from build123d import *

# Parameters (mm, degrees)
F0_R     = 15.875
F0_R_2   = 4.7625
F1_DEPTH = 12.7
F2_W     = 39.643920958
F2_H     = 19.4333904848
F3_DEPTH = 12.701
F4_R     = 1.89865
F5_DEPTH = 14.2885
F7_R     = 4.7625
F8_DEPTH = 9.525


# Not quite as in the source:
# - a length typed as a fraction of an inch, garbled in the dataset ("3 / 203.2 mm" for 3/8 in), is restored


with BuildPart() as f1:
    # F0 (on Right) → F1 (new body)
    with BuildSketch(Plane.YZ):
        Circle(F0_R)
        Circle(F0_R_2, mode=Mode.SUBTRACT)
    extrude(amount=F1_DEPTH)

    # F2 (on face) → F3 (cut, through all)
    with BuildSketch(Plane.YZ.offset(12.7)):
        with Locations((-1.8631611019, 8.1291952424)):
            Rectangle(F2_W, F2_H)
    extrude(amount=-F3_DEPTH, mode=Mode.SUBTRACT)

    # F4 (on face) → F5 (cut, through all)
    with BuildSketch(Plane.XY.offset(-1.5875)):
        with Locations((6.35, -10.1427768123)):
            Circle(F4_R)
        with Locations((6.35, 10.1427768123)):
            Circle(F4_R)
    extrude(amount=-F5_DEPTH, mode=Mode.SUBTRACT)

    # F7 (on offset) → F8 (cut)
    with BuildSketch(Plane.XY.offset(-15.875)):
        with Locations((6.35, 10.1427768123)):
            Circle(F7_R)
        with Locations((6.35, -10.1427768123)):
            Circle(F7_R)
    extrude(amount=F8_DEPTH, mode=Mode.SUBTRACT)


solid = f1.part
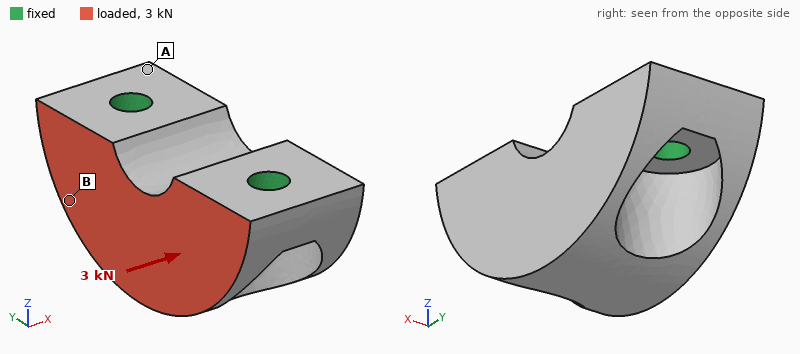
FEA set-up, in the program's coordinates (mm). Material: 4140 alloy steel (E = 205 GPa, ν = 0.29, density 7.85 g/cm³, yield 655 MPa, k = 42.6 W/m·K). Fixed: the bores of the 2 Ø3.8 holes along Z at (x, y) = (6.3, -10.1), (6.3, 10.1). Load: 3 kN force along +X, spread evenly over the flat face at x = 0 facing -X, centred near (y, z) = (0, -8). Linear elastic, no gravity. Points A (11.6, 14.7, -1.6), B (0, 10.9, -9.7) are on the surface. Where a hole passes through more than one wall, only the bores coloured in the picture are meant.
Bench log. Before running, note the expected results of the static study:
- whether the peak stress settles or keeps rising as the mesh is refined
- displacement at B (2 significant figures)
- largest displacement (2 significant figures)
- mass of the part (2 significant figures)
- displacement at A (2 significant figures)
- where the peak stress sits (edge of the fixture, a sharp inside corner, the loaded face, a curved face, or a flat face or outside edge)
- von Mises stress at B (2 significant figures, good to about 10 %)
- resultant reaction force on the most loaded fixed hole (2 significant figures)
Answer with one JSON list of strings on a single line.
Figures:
["keeps rising", "6.9 µm", "11 µm", "25 g", "1.7 µm", "edge of the fixture", "31 MPa", "1.5 kN"]
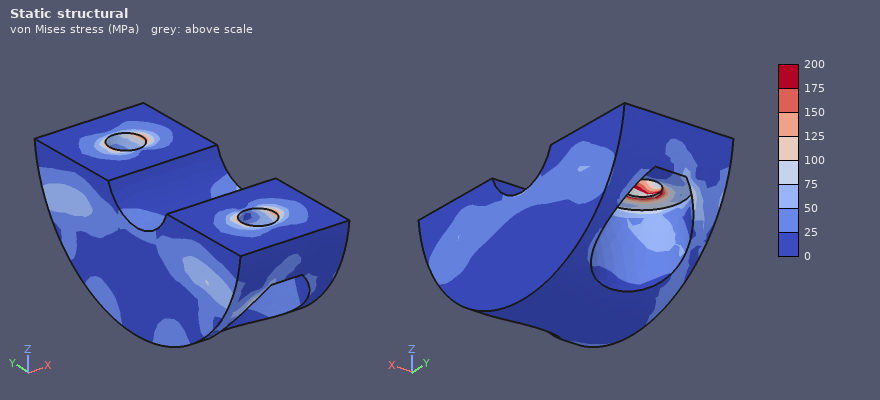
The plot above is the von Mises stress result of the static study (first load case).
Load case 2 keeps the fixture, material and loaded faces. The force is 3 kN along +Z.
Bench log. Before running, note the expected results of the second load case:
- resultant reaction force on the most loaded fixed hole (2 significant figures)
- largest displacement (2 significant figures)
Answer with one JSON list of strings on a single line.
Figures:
["1.6 kN", "13 µm"]
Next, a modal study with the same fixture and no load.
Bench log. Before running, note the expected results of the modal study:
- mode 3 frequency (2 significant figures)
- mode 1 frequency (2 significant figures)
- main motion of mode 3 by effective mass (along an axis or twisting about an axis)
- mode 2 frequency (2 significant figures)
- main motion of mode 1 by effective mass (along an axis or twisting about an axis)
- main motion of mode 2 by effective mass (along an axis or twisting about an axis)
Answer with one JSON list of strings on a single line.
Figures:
["44 kHz", "20 kHz", "along Y", "41 kHz", "along X", "along Z"]
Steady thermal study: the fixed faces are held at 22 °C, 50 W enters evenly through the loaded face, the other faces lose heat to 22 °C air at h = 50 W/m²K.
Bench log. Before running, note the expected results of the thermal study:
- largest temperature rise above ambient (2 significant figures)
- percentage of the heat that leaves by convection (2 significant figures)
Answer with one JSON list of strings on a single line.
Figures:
["68 K", "4.3 %"]
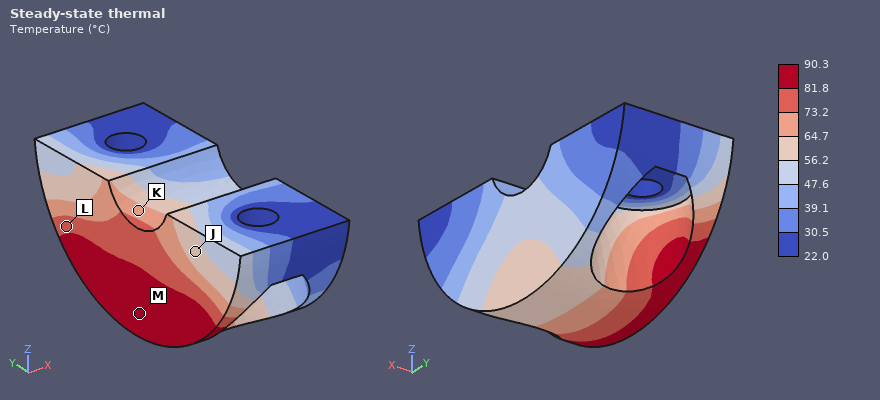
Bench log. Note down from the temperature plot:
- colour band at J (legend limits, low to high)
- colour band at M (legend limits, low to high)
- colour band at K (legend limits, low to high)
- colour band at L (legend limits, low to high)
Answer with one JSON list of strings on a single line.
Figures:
["56.2 to 64.7 °C", "81.8 to 90.3 °C", "64.7 to 73.2 °C", "73.2 to 81.8 °C"]
